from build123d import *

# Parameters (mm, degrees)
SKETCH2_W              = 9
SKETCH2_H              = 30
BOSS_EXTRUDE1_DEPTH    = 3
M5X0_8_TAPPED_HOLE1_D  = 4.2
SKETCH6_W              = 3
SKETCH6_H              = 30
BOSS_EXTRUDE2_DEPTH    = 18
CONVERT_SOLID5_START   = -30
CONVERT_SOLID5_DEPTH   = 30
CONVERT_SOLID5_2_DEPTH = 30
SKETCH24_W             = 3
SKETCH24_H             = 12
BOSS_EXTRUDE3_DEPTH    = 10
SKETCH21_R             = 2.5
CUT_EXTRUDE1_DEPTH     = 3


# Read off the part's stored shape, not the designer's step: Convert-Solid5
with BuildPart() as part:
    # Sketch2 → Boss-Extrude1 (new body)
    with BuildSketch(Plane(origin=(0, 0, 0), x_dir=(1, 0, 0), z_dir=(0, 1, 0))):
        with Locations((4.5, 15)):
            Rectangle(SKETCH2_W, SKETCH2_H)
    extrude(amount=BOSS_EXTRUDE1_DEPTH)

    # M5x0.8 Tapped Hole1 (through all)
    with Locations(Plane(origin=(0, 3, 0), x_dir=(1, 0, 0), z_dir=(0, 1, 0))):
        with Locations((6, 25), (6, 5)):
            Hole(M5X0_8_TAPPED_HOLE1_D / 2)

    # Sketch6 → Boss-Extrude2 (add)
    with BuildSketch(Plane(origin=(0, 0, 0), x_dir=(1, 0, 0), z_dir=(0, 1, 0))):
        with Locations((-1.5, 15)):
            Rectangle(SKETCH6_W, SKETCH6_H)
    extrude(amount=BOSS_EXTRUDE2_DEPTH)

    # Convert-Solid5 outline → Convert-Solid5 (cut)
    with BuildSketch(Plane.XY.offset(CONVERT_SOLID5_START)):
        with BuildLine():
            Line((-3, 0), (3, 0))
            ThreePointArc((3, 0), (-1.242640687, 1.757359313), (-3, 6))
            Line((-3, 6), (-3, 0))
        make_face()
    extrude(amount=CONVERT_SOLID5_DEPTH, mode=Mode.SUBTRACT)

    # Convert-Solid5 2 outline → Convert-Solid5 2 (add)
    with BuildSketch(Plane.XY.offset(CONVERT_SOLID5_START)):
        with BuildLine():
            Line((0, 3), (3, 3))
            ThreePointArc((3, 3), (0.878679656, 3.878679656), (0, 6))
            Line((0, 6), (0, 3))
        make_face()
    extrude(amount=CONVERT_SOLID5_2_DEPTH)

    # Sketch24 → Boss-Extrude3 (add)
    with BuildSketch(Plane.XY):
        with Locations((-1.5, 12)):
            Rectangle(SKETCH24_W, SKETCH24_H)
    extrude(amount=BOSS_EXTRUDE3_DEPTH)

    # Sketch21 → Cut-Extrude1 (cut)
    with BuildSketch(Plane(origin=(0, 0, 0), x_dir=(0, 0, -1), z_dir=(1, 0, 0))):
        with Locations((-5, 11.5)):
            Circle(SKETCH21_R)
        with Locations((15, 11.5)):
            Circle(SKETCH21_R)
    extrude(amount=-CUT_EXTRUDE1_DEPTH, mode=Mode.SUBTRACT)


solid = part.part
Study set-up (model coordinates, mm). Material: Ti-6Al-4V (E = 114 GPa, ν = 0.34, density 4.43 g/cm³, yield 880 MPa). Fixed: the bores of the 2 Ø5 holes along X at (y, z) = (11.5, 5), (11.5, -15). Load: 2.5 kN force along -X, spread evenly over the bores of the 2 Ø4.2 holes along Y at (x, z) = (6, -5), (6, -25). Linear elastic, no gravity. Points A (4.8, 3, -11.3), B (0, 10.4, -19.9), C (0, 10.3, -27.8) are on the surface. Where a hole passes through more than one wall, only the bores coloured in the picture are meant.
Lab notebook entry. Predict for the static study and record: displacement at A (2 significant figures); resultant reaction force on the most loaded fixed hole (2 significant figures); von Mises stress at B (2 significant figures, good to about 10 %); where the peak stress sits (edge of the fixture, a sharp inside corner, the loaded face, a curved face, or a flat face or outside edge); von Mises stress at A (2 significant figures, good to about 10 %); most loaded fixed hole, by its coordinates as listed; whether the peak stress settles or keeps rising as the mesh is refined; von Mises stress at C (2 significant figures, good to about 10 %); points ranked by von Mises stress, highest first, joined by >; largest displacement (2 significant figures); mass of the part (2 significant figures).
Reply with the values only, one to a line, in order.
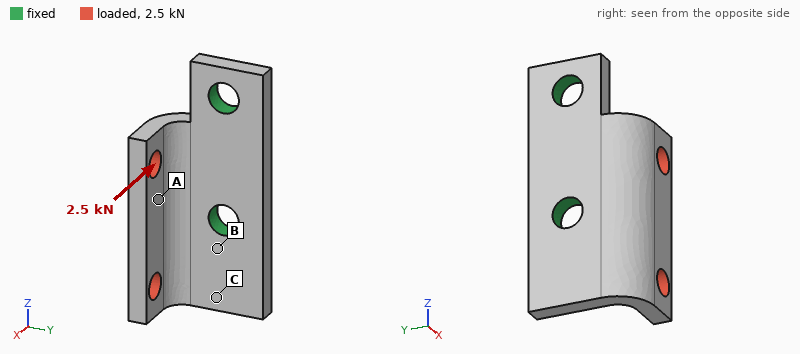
0.12 mm
2.3 kN
310 MPa
edge of the fixture
84 MPa
(11.5, -15)
keeps rising
160 MPa
B > C > A
0.26 mm
11 g
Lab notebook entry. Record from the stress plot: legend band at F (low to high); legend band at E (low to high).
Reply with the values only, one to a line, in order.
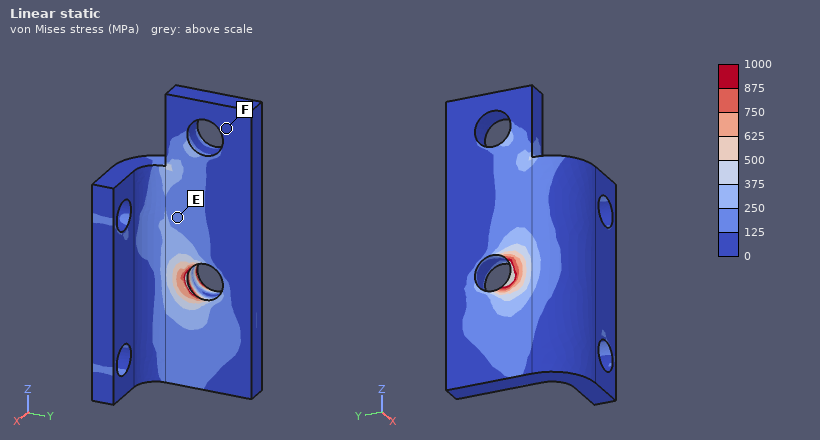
0 to 125 MPa
125 to 250 MPa
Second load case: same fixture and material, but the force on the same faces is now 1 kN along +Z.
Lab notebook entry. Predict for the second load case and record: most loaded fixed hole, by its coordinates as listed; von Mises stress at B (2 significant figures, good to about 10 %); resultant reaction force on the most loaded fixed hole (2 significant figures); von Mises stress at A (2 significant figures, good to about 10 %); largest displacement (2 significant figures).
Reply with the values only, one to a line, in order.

(11.5, -15)
74 MPa
820 N
58 MPa
62 µm
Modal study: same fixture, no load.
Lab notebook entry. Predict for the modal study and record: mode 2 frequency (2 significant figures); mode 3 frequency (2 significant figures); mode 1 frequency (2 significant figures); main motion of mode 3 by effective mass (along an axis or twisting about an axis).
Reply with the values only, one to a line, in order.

11 kHz
17 kHz
8800 Hz
along X
